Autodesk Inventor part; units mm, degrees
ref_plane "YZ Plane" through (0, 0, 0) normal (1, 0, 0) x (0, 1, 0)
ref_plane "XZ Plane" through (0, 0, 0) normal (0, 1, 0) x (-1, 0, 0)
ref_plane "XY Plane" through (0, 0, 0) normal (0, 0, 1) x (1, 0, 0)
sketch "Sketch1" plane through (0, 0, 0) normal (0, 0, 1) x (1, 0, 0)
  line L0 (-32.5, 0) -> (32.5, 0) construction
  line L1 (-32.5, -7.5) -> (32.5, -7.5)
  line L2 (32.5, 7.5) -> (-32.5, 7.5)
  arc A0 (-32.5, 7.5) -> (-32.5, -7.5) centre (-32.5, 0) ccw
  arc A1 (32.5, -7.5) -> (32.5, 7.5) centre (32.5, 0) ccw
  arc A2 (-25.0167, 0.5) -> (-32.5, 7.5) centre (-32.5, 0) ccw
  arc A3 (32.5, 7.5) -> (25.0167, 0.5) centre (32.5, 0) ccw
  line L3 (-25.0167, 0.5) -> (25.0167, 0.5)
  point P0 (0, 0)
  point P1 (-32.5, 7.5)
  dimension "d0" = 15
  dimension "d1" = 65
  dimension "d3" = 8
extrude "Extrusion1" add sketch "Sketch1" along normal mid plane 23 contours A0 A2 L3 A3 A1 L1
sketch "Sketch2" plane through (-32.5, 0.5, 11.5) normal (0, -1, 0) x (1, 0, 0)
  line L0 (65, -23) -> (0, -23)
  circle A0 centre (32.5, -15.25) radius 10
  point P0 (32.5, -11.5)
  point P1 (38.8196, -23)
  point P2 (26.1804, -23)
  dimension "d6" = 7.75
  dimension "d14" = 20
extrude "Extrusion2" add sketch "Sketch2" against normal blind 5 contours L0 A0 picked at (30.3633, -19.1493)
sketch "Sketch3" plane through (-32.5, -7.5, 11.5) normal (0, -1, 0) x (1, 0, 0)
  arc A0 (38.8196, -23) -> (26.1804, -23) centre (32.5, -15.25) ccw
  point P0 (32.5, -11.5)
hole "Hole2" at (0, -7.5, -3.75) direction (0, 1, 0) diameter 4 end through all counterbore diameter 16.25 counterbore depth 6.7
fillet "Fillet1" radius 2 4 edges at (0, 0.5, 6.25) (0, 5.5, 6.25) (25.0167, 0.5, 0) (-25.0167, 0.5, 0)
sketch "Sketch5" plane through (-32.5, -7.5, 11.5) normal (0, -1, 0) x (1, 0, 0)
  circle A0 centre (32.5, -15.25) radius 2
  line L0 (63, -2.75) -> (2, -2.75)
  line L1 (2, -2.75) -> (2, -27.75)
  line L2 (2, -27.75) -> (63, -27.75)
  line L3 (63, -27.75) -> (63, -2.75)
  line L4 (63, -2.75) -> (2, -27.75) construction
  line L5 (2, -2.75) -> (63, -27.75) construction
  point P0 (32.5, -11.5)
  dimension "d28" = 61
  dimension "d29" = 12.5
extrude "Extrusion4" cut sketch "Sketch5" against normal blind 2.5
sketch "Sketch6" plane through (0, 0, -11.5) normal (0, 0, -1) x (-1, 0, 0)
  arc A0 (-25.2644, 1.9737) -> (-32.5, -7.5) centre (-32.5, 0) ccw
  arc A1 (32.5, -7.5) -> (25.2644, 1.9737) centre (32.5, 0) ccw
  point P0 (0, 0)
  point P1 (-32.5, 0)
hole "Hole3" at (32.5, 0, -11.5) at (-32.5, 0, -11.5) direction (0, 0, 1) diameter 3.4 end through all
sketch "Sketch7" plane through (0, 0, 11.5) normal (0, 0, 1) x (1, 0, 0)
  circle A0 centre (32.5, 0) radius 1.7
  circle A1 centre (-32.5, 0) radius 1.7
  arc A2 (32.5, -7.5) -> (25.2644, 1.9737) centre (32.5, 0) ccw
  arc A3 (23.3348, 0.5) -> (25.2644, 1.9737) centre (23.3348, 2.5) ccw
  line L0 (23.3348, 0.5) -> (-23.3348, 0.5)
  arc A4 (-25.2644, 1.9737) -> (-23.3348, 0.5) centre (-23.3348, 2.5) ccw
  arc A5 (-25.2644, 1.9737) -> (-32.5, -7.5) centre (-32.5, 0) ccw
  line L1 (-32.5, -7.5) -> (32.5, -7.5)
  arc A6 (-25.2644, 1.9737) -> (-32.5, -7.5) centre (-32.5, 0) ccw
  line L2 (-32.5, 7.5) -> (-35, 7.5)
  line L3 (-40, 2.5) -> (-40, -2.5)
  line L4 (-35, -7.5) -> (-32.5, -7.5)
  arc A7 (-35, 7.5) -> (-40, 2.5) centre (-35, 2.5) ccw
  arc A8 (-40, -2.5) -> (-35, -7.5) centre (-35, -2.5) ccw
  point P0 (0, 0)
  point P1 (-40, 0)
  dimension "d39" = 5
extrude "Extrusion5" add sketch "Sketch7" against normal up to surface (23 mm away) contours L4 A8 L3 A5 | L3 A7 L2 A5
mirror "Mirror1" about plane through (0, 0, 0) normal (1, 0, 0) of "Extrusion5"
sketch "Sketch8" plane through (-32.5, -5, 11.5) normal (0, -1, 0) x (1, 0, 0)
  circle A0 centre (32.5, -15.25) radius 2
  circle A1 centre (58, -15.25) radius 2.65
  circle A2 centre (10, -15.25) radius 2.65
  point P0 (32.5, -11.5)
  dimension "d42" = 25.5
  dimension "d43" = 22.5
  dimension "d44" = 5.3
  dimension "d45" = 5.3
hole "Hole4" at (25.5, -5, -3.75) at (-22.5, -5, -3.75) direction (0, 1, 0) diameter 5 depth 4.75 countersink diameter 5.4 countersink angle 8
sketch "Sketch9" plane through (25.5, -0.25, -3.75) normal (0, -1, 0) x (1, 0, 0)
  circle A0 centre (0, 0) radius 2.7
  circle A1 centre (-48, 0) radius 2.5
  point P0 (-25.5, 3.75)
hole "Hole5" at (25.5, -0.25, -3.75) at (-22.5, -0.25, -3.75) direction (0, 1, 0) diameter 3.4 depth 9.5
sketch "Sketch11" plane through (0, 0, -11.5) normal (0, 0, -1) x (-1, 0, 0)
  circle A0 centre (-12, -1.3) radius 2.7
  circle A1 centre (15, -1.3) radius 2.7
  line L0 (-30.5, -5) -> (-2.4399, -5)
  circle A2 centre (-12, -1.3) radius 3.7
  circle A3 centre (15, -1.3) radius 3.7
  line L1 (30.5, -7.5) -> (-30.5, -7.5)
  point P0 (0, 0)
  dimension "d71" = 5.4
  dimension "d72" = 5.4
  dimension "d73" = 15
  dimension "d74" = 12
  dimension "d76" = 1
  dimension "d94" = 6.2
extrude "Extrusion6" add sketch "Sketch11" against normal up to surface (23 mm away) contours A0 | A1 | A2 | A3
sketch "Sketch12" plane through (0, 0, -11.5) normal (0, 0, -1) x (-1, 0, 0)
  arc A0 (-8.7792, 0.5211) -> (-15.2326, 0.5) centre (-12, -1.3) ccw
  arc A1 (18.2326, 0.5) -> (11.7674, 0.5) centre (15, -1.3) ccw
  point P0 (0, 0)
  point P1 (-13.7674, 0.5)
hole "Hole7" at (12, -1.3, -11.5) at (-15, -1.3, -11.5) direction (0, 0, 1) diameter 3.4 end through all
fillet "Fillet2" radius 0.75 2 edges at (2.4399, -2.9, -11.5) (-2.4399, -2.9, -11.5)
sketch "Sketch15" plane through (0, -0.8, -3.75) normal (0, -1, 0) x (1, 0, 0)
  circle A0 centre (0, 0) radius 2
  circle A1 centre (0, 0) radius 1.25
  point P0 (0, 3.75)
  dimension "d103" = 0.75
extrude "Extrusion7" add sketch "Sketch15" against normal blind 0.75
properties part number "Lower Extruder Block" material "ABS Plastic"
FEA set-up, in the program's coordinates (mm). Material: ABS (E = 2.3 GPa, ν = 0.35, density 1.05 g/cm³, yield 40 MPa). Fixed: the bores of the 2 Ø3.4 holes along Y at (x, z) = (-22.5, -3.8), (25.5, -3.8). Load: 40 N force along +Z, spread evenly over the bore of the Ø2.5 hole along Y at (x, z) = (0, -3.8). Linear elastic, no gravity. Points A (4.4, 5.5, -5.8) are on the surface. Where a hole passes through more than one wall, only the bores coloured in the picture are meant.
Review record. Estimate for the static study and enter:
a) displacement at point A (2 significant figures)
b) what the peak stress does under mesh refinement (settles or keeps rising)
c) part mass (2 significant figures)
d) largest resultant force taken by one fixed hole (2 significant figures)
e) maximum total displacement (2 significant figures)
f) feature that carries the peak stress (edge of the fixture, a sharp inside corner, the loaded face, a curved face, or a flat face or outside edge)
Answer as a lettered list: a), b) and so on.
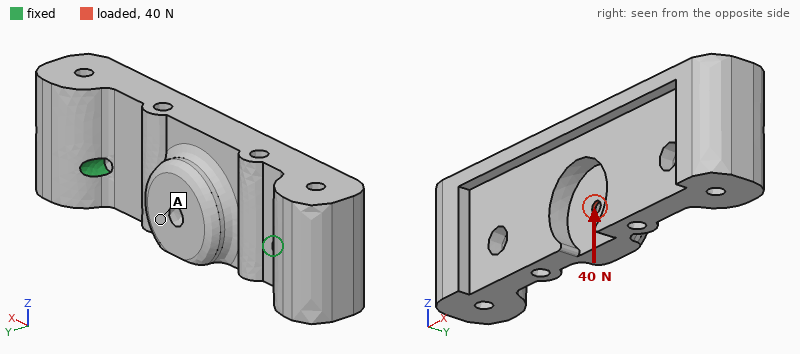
a) 21 µm
b) keeps rising
c) 16 g
d) 23 N
e) 29 µm
f) a sharp inside corner
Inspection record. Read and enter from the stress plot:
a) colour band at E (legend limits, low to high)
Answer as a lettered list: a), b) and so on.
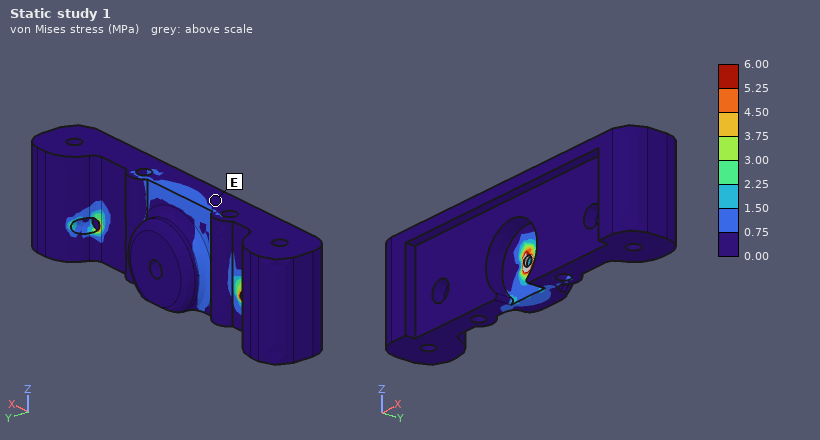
a) 0.00 to 0.75 MPa
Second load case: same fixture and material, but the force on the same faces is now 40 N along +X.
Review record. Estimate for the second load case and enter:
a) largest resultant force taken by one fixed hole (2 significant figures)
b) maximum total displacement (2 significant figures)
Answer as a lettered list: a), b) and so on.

a) 20 N
b) 13 µm
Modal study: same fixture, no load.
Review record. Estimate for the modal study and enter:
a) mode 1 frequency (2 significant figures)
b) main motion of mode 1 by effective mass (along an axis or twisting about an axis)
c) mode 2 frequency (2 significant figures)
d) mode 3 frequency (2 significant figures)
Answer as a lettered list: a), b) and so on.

a) 1100 Hz
b) along Y
c) 1400 Hz
d) 2300 Hz
